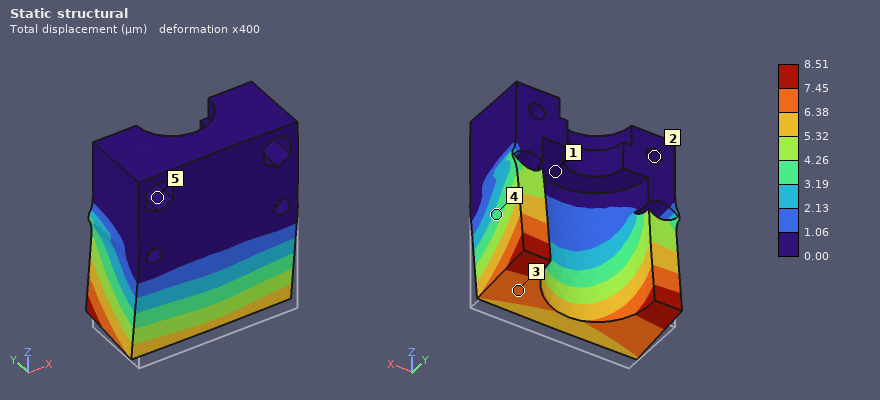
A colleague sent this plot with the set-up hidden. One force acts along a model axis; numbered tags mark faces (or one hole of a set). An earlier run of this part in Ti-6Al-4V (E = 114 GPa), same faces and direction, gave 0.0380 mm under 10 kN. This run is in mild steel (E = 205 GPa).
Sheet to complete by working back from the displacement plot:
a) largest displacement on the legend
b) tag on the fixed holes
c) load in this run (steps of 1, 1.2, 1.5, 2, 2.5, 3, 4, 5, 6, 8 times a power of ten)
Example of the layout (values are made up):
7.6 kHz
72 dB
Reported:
8.51 µm
2
4 kN
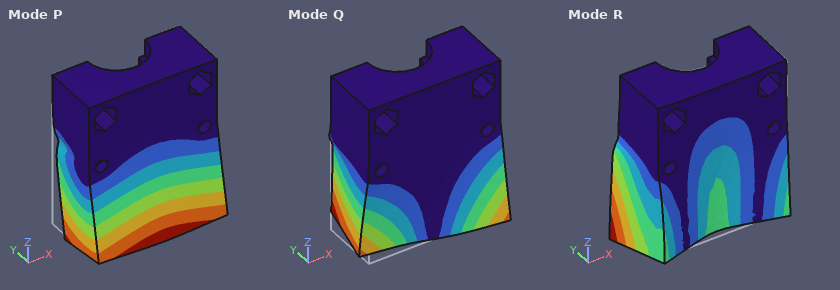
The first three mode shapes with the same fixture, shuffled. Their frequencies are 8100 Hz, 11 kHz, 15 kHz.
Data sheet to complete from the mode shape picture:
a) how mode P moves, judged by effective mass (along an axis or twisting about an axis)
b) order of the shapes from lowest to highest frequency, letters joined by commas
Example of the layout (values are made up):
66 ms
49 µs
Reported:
along Y
P, Q, R
